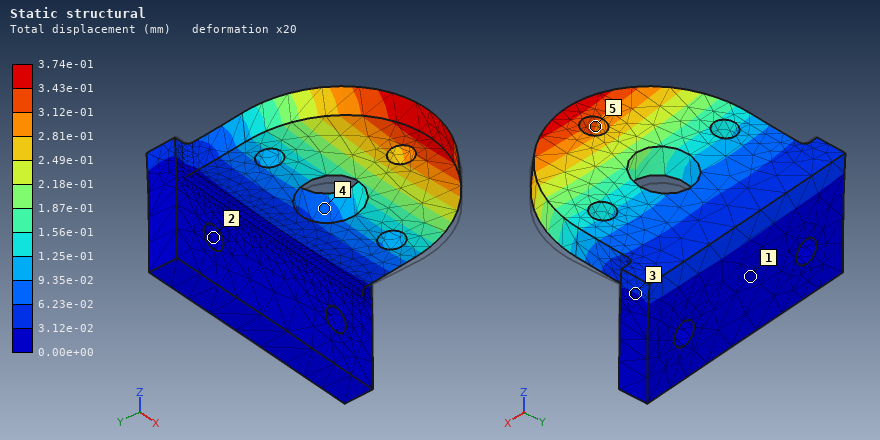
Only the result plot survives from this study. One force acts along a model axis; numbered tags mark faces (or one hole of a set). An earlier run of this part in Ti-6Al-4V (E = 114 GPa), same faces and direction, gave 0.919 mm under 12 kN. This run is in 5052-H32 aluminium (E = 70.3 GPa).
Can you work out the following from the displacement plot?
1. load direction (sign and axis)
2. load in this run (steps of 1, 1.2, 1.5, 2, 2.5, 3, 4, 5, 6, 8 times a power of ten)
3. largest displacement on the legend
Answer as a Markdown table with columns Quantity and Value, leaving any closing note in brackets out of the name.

| Quantity | Value |
|---|---|
| load direction | +Z |
| load in this run | 3 kN |
| largest displacement on the legend | 3.74e-01 mm |
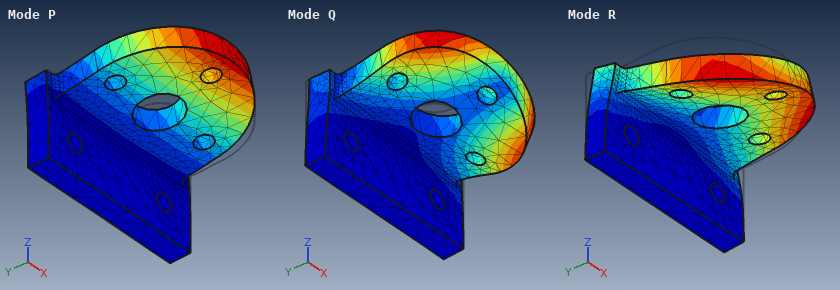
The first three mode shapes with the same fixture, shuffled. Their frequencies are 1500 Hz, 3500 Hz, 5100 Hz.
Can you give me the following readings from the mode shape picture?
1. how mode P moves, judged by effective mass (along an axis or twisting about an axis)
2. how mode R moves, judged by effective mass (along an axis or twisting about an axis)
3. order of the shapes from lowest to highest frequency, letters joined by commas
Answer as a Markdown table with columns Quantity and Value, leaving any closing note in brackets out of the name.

| Quantity | Value |
|---|---|
| how mode P moves, judged by effective mass | along Z |
| how mode R moves, judged by effective mass | along X |
| order of the shapes from lowest to highest frequency, letters joined by commas | P, R, Q |
